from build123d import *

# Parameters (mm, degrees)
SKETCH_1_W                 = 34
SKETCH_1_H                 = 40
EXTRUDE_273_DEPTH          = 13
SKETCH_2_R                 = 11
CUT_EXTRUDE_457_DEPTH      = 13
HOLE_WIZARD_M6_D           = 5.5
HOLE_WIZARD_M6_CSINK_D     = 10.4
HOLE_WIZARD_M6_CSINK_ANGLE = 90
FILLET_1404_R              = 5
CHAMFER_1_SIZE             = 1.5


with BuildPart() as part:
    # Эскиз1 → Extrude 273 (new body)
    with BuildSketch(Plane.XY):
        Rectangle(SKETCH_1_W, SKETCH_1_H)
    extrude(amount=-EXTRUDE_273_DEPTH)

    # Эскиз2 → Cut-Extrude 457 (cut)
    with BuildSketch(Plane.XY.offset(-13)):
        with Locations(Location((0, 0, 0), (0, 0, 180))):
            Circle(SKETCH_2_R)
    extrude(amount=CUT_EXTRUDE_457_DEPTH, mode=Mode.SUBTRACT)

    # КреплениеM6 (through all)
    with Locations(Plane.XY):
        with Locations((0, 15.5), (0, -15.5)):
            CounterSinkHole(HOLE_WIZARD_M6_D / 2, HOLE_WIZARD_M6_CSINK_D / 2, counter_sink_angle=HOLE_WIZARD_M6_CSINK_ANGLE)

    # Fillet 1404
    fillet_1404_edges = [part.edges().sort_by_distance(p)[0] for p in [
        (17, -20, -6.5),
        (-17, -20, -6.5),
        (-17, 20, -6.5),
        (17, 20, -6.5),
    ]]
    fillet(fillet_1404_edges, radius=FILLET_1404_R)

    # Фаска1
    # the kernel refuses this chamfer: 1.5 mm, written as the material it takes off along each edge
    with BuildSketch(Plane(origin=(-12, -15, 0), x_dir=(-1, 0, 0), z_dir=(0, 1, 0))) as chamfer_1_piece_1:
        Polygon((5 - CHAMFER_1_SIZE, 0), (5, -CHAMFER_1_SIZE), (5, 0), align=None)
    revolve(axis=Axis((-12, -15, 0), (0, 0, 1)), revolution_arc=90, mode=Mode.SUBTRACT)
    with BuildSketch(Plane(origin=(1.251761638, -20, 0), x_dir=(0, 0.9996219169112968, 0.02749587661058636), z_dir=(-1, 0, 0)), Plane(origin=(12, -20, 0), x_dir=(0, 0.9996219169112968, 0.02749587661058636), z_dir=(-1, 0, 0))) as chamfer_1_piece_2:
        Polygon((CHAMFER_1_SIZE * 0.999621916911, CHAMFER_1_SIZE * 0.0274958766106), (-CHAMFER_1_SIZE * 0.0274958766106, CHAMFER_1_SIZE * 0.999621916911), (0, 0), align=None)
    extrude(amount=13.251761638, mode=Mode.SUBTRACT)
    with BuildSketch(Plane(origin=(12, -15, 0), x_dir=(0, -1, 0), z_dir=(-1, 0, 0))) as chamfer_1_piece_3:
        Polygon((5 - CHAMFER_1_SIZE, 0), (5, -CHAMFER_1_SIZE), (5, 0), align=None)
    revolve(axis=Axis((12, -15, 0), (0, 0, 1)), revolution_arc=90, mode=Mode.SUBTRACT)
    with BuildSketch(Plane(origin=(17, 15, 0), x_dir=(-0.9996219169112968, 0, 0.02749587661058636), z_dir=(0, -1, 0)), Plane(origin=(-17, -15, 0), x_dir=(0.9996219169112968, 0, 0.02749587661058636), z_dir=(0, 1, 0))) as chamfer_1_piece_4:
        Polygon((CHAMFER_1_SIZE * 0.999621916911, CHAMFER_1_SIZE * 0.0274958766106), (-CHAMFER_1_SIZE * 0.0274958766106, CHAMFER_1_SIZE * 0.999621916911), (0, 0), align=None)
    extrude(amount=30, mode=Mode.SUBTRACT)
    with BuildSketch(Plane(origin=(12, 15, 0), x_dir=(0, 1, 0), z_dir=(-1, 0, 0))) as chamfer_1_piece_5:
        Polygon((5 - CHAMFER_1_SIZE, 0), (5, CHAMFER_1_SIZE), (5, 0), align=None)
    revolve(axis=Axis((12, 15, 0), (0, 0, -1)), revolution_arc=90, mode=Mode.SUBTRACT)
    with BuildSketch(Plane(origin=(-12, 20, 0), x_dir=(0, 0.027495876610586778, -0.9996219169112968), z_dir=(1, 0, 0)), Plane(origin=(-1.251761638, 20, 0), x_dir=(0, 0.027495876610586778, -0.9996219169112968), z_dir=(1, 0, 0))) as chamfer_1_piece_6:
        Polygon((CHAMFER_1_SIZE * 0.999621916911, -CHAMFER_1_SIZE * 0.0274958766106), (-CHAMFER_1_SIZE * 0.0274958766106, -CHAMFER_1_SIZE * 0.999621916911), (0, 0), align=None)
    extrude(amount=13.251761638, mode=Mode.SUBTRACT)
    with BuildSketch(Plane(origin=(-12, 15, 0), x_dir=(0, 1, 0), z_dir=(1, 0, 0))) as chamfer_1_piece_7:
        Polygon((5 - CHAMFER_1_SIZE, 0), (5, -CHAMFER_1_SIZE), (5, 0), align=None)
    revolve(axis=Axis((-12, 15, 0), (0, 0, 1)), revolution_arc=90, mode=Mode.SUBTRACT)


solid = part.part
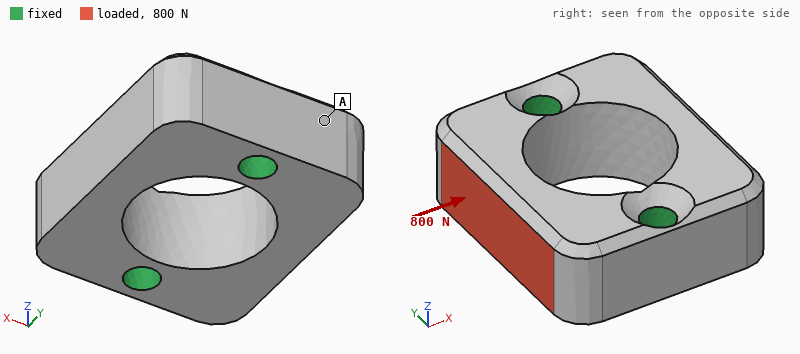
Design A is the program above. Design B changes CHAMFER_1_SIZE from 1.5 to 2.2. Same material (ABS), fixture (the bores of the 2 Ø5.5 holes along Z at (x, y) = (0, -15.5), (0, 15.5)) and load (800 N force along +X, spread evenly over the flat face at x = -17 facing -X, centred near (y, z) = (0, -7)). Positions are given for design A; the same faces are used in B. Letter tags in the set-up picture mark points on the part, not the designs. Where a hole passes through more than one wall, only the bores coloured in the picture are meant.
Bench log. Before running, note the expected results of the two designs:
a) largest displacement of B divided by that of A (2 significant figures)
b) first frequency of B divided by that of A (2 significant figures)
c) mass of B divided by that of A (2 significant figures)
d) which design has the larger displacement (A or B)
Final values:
1.1
1.0
0.99
B
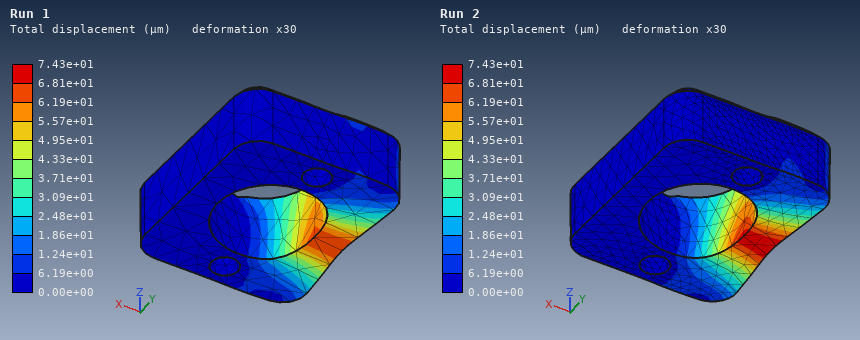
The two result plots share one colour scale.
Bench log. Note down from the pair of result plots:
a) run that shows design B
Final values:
Run 2
